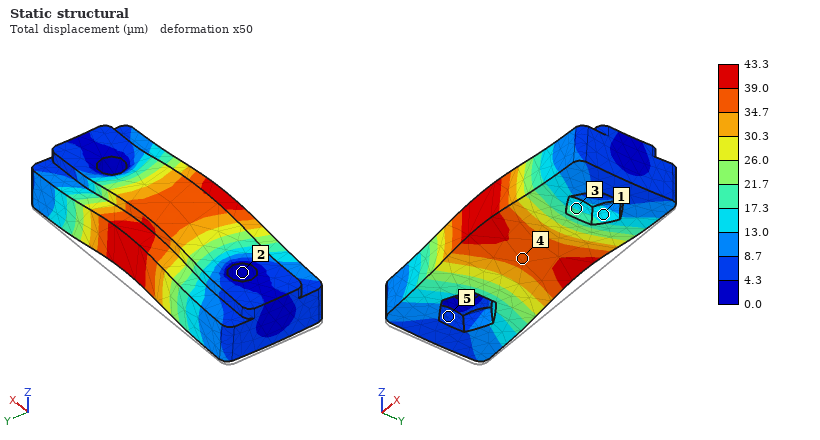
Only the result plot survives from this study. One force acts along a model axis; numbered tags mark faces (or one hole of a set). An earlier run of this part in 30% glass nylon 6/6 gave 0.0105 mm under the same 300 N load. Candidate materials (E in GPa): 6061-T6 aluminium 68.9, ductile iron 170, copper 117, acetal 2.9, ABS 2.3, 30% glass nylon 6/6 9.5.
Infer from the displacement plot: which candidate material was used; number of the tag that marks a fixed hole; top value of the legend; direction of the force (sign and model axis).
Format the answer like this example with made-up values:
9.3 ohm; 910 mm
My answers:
ABS; 2; 43.3 µm; +Z
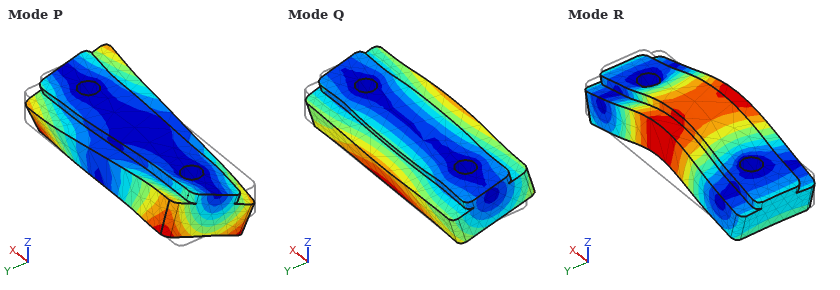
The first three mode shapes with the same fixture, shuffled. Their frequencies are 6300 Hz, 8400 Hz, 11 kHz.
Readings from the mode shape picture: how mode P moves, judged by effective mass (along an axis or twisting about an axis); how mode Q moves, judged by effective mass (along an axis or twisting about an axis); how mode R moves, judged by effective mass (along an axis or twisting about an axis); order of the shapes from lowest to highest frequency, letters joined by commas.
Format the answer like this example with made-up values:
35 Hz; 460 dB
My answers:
twisting about Z; along Y; along Z; Q, R, P
